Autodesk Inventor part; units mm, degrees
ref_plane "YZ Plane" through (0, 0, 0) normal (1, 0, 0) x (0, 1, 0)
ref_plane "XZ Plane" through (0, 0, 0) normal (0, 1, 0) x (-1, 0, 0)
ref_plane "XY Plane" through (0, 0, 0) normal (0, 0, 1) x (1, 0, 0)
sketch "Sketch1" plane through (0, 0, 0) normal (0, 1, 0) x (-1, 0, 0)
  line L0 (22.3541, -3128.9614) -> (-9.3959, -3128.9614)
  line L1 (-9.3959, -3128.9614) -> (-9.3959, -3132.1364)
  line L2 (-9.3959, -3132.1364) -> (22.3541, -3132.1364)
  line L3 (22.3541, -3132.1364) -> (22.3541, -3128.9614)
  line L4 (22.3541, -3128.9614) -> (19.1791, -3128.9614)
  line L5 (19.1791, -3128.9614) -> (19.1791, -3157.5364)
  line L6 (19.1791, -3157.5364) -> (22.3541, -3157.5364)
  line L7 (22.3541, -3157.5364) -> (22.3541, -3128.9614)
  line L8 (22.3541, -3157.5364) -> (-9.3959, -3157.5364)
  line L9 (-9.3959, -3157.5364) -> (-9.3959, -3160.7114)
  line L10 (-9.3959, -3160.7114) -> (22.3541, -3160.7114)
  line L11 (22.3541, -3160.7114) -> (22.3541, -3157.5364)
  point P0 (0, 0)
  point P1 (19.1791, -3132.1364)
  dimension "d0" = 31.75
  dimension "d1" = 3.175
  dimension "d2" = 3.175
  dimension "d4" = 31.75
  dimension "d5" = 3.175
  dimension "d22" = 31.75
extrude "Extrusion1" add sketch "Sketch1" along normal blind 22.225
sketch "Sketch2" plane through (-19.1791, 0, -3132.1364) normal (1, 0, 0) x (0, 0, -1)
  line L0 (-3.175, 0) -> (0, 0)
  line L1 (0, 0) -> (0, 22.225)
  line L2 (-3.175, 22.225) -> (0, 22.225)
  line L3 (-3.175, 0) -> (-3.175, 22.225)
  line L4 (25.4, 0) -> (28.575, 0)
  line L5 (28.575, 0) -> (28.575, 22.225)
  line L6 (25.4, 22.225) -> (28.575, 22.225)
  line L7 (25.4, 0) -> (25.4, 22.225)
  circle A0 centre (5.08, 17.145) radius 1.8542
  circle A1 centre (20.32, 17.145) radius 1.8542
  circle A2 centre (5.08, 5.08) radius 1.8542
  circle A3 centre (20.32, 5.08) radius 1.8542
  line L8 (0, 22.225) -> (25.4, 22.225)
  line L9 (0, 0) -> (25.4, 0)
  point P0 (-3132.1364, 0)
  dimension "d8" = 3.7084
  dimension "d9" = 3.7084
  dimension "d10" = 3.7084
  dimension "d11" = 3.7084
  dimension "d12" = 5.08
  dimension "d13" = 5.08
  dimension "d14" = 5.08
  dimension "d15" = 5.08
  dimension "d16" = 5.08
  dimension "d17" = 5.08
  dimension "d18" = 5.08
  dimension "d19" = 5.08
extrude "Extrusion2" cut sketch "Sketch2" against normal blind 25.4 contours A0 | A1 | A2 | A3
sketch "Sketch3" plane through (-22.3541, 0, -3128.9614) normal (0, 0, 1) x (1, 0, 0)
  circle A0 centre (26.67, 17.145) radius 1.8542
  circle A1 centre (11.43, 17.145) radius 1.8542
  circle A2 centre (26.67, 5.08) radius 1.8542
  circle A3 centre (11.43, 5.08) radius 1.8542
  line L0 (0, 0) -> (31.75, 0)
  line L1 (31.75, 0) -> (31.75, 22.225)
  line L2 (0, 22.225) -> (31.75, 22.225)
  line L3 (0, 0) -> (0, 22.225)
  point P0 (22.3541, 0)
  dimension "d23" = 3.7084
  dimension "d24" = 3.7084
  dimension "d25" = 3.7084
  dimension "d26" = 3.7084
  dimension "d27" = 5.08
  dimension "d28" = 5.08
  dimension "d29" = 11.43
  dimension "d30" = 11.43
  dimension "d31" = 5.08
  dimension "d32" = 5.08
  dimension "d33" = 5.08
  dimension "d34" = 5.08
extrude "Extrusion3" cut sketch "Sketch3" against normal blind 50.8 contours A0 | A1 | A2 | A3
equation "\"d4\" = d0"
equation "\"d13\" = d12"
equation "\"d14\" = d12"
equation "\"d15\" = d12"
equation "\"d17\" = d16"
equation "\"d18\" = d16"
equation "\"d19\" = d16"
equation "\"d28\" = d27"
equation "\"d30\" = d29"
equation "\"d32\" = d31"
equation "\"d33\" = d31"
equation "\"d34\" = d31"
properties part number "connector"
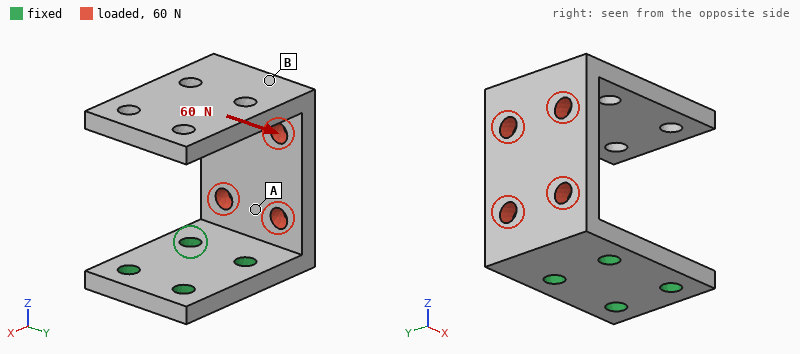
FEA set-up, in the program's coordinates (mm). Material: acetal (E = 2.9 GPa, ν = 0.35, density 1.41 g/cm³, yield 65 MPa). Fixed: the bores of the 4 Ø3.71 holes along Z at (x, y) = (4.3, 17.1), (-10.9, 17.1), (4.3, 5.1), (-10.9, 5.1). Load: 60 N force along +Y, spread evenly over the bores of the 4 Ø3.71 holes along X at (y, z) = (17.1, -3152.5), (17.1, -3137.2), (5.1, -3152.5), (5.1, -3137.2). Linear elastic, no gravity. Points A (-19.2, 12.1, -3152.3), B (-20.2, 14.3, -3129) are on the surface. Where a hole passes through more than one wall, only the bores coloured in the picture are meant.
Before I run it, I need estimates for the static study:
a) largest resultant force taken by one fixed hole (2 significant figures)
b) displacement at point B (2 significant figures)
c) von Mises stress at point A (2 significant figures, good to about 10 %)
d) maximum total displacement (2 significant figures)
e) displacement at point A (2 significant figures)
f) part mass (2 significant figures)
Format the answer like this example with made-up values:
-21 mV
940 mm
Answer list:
73 N
0.39 mm
4.6 MPa
0.60 mm
0.099 mm
8.3 g
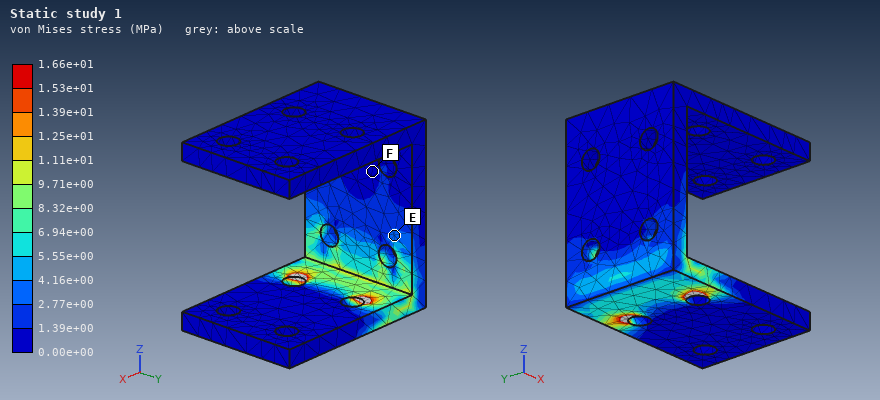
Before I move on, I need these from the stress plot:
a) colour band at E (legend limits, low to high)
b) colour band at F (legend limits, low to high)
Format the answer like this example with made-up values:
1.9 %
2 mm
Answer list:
2.77e+00 to 4.16e+00 MPa
0.00e+00 to 1.39e+00 MPa
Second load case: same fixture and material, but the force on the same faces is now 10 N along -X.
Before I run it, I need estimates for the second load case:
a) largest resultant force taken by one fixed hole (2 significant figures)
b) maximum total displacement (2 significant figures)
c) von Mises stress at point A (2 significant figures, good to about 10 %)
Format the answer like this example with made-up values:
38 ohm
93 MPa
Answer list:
5.0 N
0.55 mm
2.6 MPa
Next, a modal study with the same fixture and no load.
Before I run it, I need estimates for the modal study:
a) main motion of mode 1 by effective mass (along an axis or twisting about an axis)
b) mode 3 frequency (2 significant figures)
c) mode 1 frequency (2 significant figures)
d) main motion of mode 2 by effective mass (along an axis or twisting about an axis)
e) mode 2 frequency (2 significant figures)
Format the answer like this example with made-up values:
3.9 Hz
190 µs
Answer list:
along X
650 Hz
240 Hz
along Y
400 Hz
